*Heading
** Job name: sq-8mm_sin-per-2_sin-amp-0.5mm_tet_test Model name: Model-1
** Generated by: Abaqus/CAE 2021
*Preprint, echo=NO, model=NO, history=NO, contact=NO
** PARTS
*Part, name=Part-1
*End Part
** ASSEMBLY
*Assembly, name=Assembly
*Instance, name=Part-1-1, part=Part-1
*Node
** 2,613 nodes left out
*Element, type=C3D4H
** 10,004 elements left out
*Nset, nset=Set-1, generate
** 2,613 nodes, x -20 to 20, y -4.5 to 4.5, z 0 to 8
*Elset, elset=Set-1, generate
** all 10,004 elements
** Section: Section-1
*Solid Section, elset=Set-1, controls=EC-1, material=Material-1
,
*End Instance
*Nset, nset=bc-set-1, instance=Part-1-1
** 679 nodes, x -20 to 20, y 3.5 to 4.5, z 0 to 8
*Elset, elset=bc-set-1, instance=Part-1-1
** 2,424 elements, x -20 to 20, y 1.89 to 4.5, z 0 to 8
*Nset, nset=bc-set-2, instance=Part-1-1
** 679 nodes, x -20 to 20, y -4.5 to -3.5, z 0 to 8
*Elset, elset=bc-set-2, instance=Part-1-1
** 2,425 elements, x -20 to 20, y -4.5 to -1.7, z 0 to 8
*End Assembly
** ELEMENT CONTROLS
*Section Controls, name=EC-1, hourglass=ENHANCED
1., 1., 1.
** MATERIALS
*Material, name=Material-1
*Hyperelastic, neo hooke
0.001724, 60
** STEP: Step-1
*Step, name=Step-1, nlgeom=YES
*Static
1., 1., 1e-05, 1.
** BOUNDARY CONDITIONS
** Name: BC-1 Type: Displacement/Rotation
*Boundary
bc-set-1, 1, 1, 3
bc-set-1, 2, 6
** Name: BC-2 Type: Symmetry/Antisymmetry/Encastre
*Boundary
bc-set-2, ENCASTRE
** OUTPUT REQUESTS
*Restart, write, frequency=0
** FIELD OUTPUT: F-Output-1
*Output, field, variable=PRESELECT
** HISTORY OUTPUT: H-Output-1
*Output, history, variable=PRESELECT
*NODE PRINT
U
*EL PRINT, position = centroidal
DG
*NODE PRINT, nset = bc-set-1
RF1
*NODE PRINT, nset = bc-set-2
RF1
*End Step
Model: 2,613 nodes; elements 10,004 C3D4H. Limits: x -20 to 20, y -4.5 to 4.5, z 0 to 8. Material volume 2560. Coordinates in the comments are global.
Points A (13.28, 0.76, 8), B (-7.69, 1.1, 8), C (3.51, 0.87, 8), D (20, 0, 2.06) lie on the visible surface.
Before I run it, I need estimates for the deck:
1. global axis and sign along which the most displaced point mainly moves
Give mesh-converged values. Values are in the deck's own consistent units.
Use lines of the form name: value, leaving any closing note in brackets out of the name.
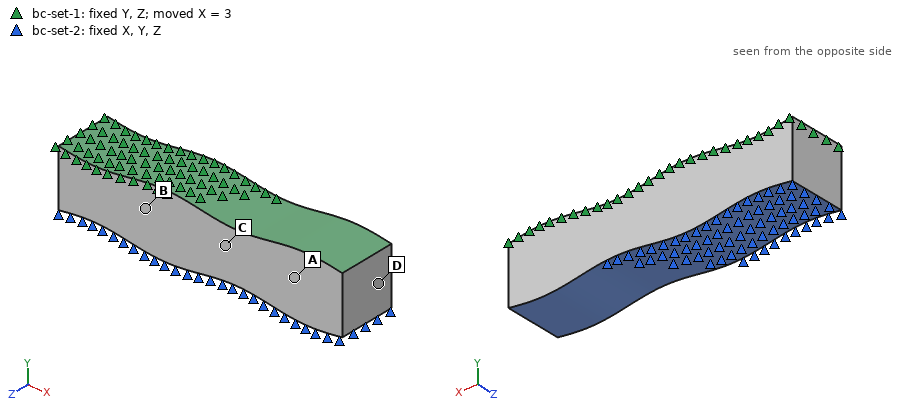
global axis and sign along which the most displaced point mainly moves: +X
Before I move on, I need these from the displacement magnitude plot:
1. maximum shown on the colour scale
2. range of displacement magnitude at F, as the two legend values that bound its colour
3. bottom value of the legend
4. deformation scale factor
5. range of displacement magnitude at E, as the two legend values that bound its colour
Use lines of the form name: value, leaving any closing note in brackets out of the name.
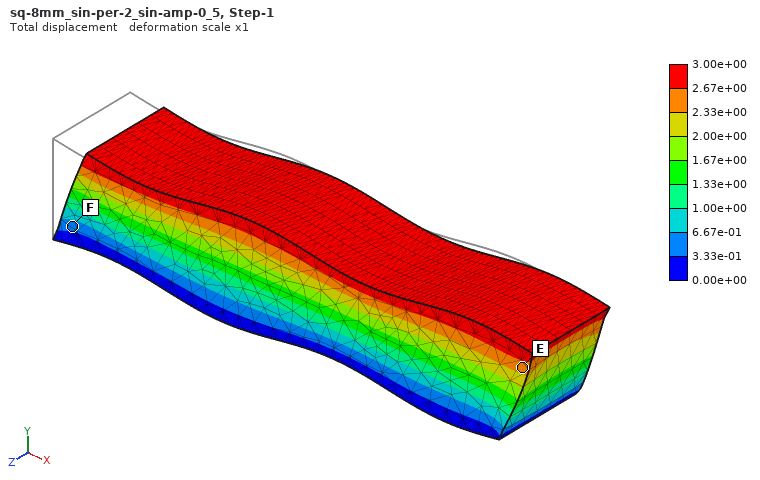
maximum shown on the colour scale: 3.00e+00
range of displacement magnitude at F, as the two legend values that bound its colour: 3.33e-01 to 6.67e-01
bottom value of the legend: 0.00e+00
deformation scale factor: 1
range of displacement magnitude at E, as the two legend values that bound its colour: 2.33e+00 to 2.67e+00
